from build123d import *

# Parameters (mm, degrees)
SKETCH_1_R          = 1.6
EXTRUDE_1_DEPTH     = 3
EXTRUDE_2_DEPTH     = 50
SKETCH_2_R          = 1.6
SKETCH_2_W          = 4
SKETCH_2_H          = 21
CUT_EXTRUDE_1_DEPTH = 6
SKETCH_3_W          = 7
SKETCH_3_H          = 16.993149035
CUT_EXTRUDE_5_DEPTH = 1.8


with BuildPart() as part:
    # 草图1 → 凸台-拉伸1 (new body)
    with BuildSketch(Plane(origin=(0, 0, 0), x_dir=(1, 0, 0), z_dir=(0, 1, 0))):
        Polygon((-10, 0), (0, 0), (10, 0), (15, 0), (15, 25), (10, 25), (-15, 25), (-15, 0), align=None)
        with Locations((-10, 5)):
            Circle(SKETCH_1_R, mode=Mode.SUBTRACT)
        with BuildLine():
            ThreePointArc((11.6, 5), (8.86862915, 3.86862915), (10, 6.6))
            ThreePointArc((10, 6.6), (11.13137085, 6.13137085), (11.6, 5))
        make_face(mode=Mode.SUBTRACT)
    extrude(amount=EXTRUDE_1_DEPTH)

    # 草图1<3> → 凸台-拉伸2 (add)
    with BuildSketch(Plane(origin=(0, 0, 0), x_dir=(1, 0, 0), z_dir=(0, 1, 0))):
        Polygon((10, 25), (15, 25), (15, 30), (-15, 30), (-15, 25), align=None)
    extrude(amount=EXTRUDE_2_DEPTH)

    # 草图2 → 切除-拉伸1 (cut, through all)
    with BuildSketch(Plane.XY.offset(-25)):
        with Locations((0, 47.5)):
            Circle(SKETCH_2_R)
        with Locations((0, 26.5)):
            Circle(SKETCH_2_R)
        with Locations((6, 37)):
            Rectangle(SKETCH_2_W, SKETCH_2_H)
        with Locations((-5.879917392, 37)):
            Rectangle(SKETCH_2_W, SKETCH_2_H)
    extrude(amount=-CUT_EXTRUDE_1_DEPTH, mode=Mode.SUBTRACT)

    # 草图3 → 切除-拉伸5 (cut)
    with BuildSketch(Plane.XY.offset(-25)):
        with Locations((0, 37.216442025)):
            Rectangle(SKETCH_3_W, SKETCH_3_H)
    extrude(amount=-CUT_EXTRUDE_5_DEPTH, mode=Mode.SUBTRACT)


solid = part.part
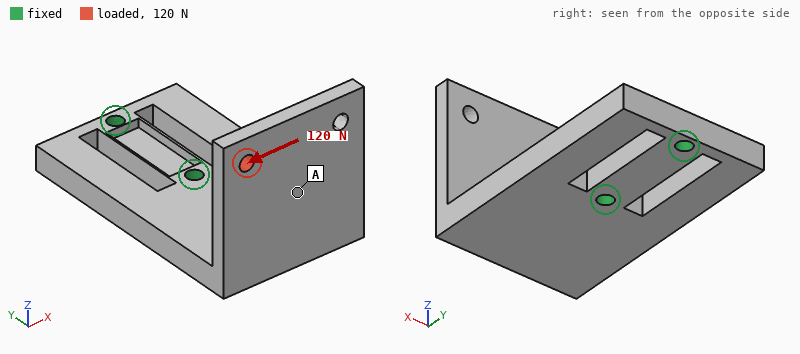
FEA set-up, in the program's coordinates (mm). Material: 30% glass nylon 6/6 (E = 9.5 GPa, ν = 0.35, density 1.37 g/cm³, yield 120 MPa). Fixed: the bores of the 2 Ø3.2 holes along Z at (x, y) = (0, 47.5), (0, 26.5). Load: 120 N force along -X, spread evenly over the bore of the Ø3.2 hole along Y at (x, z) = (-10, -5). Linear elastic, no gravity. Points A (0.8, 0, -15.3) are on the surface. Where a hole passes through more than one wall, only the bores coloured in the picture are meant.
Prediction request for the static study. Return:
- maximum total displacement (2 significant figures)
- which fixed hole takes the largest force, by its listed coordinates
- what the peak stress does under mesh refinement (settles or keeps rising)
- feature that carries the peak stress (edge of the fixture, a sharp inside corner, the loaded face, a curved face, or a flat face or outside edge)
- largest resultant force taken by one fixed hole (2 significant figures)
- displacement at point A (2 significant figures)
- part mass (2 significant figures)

0.74 mm
(0, 26.5)
keeps rising
edge of the fixture
200 N
0.33 mm
12 g
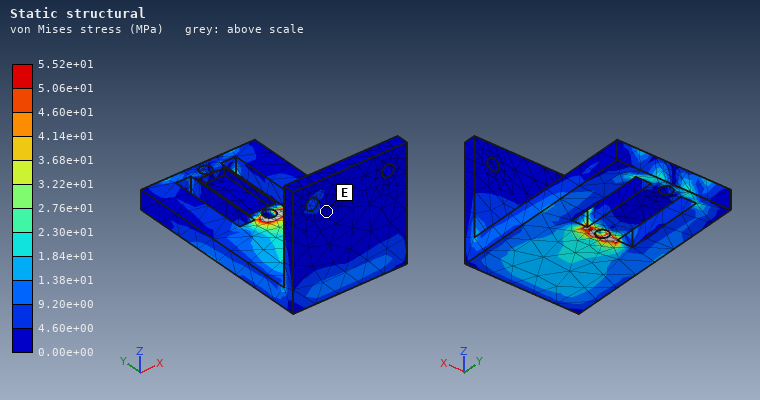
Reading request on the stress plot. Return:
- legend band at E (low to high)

0.00e+00 to 4.60e+00 MPa
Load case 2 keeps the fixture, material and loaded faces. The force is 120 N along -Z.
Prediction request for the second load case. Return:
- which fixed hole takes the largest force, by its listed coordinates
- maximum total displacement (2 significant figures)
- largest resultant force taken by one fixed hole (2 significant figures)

(0, 26.5)
0.70 mm
170 N
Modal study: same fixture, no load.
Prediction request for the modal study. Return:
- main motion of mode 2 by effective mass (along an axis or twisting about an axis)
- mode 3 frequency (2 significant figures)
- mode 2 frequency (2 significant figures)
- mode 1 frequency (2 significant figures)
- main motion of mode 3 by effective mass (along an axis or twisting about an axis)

along X
2300 Hz
1500 Hz
1100 Hz
along Z
